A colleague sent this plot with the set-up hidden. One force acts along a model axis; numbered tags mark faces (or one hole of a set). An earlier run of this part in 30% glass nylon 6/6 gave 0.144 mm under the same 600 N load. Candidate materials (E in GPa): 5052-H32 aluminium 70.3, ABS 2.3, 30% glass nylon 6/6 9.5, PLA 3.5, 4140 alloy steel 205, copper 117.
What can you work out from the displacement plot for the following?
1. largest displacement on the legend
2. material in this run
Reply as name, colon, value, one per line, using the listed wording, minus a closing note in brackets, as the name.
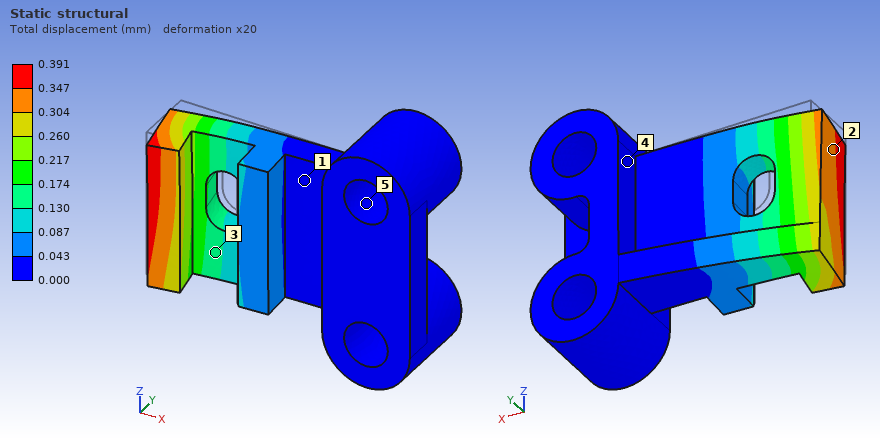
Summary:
largest displacement on the legend: 0.391 mm
material in this run: PLA
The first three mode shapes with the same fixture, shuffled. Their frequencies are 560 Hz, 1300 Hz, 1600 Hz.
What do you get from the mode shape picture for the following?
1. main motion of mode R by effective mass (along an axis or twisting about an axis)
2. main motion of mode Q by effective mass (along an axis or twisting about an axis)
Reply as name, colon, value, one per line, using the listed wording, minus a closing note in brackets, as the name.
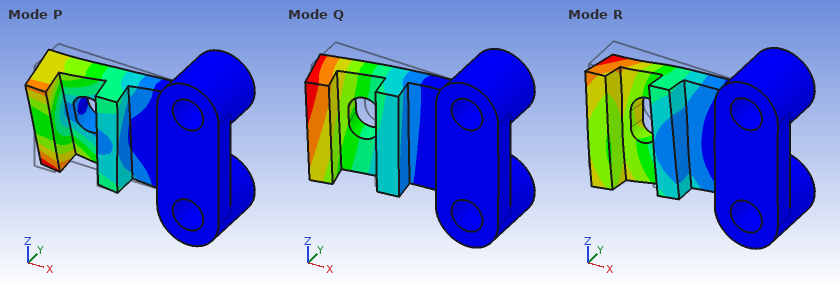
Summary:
main motion of mode R by effective mass: along Z
main motion of mode Q by effective mass: along Y
